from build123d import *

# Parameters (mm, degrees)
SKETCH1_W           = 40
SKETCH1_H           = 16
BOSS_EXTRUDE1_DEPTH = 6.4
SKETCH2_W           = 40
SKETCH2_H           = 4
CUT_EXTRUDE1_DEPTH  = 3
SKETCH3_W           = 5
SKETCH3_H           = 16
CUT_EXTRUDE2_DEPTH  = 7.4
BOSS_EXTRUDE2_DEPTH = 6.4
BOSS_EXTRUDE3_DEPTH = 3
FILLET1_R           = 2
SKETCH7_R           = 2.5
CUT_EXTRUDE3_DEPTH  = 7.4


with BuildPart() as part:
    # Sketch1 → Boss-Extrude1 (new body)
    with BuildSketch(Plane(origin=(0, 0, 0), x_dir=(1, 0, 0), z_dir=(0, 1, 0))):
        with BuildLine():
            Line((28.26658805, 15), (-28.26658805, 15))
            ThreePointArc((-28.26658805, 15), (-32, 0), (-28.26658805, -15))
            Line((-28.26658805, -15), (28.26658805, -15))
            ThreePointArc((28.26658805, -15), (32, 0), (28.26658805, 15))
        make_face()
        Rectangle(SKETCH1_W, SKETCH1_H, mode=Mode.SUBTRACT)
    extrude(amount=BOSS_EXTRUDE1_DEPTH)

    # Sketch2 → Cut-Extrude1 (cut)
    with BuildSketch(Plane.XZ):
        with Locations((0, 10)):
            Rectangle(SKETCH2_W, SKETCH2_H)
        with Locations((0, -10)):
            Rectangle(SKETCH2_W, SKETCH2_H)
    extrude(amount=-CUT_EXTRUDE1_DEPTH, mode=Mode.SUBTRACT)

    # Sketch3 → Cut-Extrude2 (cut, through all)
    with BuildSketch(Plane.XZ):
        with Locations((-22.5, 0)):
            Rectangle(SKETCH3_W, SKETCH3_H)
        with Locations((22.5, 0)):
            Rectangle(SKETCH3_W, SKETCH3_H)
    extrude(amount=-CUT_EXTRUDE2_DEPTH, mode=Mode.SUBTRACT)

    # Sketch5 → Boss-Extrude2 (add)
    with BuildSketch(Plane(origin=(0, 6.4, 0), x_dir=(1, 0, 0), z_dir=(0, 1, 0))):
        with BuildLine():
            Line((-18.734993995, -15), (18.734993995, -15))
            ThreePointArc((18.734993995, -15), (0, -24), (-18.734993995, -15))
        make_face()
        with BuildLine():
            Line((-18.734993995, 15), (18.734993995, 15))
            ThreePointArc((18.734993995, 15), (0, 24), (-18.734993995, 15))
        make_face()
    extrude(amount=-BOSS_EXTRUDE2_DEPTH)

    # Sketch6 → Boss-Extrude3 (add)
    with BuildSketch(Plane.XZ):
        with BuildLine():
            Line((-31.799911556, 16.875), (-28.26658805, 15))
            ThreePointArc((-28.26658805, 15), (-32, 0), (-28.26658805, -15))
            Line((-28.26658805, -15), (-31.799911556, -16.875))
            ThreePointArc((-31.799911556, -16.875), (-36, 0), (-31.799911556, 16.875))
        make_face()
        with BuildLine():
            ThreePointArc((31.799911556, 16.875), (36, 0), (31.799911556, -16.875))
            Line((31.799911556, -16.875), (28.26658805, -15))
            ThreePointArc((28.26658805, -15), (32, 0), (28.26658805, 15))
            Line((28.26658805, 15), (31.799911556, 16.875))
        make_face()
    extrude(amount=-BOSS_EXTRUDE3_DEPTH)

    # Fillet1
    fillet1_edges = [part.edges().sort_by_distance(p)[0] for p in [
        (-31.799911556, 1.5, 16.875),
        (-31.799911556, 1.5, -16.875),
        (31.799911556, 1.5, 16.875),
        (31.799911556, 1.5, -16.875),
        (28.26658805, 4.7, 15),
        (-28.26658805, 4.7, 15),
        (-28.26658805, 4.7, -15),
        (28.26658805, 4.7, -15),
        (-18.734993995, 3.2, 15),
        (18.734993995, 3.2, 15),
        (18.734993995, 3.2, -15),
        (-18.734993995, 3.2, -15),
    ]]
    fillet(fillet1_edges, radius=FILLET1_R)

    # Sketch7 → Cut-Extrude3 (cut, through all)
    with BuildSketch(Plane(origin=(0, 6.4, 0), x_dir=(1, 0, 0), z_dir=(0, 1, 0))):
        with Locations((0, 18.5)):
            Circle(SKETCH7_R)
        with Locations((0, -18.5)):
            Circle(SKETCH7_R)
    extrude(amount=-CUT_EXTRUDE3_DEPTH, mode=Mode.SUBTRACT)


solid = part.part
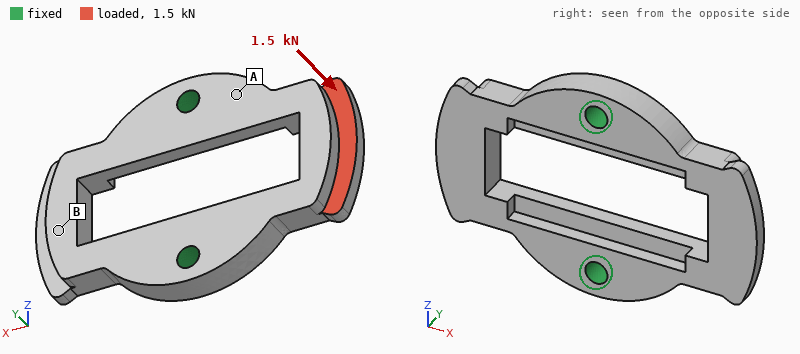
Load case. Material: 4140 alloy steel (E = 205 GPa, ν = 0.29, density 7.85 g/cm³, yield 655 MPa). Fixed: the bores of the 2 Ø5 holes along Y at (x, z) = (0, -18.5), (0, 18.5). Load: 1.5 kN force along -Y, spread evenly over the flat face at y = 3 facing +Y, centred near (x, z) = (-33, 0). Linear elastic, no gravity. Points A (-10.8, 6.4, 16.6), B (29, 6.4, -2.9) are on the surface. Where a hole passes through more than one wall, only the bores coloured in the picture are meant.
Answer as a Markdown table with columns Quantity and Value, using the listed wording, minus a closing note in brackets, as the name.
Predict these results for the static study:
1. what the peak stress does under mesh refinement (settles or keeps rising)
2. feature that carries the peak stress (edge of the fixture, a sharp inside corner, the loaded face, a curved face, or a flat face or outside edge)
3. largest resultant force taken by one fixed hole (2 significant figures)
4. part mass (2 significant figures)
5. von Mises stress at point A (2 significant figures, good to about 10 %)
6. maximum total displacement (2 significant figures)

| Quantity | Value |
|---|---|
| what the peak stress does under mesh refinement | keeps rising |
| feature that carries the peak stress | edge of the fixture |
| largest resultant force taken by one fixed hole | 840 N |
| part mass | 73 g |
| von Mises stress at point A | 230 MPa |
| maximum total displacement | 0.26 mm |
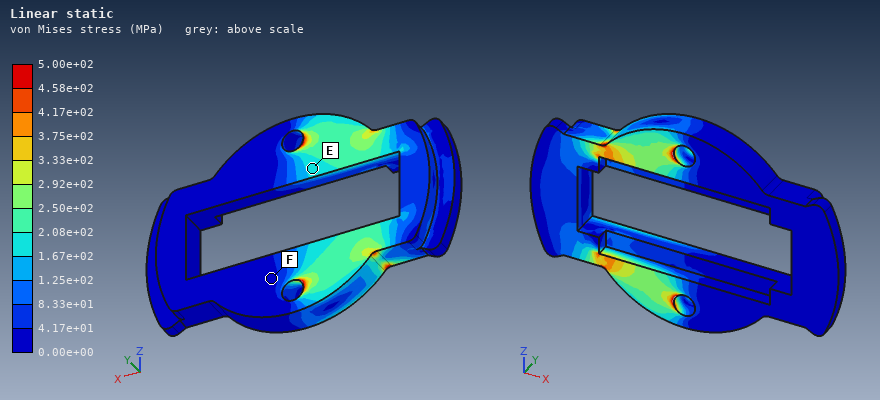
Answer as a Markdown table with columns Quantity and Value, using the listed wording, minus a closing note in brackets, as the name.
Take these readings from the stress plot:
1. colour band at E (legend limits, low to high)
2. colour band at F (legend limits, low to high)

| Quantity | Value |
|---|---|
| colour band at E | 1.67e+02 to 2.08e+02 MPa |
| colour band at F | 0.00e+00 to 4.17e+01 MPa |
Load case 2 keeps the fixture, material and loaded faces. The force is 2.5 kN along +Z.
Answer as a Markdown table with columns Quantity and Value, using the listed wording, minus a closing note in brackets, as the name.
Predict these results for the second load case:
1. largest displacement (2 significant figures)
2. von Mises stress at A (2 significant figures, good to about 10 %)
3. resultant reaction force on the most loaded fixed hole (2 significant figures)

| Quantity | Value |
|---|---|
| largest displacement | 31 µm |
| von Mises stress at A | 56 MPa |
| resultant reaction force on the most loaded fixed hole | 1.9 kN |
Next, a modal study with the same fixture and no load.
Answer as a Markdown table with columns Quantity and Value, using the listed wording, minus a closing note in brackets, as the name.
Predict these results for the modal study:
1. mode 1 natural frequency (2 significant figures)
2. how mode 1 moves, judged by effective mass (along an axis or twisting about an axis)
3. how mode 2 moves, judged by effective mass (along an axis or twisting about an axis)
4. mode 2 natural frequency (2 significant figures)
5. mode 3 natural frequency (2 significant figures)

| Quantity | Value |
|---|---|
| mode 1 natural frequency | 4100 Hz |
| how mode 1 moves, judged by effective mass | twisting about Z |
| how mode 2 moves, judged by effective mass | along Y |
| mode 2 natural frequency | 4400 Hz |
| mode 3 natural frequency | 9800 Hz |
